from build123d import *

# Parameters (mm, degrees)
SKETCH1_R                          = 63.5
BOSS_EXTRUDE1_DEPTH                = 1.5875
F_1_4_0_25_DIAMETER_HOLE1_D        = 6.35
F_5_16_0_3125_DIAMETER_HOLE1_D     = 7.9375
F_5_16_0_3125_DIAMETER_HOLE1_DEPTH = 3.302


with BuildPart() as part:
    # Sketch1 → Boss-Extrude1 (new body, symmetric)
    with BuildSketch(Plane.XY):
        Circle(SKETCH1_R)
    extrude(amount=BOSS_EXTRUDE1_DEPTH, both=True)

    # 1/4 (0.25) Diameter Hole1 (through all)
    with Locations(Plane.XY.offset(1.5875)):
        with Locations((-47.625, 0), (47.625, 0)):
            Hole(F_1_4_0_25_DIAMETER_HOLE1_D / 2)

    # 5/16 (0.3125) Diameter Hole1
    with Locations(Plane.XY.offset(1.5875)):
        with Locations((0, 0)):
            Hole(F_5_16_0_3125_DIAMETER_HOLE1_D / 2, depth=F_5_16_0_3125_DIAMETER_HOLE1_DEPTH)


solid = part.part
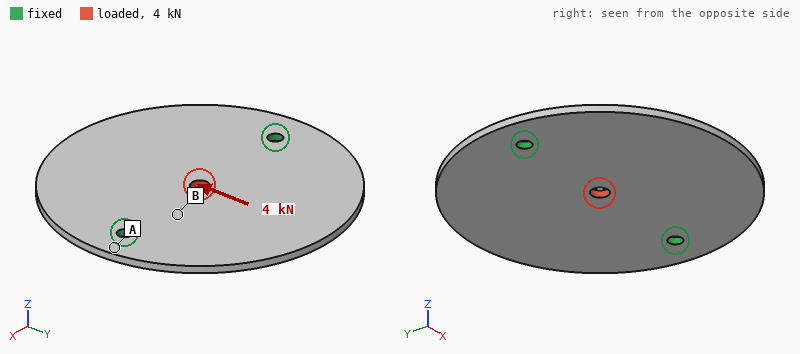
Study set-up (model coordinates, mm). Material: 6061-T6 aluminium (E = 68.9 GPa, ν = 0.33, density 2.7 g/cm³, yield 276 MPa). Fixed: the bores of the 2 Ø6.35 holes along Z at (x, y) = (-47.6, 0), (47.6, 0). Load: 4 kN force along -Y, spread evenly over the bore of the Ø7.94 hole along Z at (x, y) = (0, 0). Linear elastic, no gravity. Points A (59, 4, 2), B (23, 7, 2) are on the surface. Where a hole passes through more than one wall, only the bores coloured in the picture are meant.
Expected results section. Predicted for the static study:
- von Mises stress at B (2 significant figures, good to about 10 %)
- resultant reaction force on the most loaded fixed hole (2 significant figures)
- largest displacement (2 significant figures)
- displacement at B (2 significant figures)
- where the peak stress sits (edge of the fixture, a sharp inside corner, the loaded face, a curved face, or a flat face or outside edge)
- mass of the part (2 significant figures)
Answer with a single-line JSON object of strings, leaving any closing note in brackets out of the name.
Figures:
{"von Mises stress at B": "11 MPa", "resultant reaction force on the most loaded fixed hole": "2.0 kN", "largest displacement": "24 µm", "displacement at B": "12 µm", "where the peak stress sits": "the loaded face", "mass of the part": "110 g"}
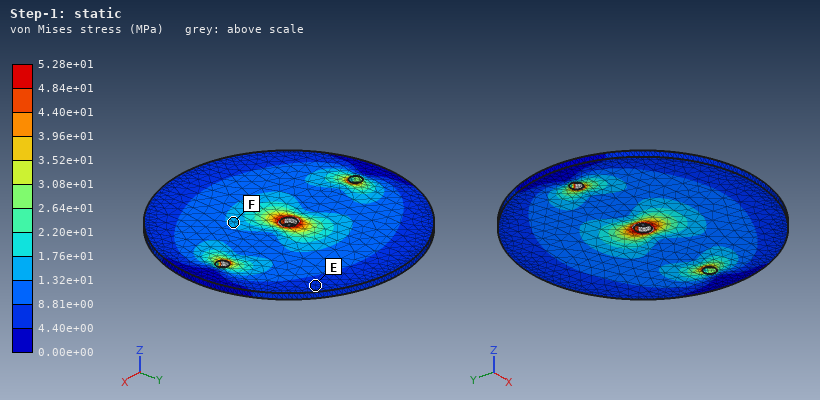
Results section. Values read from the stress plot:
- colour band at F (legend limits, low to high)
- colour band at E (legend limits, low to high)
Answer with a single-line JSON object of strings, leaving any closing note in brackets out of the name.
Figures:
{"colour band at F": "1.32e+01 to 1.76e+01 MPa", "colour band at E": "4.40e+00 to 8.81e+00 MPa"}
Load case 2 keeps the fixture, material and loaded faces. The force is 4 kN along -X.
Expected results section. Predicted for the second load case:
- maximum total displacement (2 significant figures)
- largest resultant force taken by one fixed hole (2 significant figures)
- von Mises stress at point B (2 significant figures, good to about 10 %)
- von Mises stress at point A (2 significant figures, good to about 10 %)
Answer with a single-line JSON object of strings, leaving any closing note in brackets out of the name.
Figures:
{"maximum total displacement": "18 µm", "largest resultant force taken by one fixed hole": "2.0 kN", "von Mises stress at point B": "19 MPa", "von Mises stress at point A": "9.4 MPa"}
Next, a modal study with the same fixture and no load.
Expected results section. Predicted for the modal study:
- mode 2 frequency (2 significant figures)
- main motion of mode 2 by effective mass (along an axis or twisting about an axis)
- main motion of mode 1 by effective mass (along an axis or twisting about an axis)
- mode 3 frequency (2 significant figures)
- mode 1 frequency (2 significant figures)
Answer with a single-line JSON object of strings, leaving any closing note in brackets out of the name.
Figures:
{"mode 2 frequency": "770 Hz", "main motion of mode 2 by effective mass": "along Z", "main motion of mode 1 by effective mass": "twisting about X", "mode 3 frequency": "1700 Hz", "mode 1 frequency": "600 Hz"}
